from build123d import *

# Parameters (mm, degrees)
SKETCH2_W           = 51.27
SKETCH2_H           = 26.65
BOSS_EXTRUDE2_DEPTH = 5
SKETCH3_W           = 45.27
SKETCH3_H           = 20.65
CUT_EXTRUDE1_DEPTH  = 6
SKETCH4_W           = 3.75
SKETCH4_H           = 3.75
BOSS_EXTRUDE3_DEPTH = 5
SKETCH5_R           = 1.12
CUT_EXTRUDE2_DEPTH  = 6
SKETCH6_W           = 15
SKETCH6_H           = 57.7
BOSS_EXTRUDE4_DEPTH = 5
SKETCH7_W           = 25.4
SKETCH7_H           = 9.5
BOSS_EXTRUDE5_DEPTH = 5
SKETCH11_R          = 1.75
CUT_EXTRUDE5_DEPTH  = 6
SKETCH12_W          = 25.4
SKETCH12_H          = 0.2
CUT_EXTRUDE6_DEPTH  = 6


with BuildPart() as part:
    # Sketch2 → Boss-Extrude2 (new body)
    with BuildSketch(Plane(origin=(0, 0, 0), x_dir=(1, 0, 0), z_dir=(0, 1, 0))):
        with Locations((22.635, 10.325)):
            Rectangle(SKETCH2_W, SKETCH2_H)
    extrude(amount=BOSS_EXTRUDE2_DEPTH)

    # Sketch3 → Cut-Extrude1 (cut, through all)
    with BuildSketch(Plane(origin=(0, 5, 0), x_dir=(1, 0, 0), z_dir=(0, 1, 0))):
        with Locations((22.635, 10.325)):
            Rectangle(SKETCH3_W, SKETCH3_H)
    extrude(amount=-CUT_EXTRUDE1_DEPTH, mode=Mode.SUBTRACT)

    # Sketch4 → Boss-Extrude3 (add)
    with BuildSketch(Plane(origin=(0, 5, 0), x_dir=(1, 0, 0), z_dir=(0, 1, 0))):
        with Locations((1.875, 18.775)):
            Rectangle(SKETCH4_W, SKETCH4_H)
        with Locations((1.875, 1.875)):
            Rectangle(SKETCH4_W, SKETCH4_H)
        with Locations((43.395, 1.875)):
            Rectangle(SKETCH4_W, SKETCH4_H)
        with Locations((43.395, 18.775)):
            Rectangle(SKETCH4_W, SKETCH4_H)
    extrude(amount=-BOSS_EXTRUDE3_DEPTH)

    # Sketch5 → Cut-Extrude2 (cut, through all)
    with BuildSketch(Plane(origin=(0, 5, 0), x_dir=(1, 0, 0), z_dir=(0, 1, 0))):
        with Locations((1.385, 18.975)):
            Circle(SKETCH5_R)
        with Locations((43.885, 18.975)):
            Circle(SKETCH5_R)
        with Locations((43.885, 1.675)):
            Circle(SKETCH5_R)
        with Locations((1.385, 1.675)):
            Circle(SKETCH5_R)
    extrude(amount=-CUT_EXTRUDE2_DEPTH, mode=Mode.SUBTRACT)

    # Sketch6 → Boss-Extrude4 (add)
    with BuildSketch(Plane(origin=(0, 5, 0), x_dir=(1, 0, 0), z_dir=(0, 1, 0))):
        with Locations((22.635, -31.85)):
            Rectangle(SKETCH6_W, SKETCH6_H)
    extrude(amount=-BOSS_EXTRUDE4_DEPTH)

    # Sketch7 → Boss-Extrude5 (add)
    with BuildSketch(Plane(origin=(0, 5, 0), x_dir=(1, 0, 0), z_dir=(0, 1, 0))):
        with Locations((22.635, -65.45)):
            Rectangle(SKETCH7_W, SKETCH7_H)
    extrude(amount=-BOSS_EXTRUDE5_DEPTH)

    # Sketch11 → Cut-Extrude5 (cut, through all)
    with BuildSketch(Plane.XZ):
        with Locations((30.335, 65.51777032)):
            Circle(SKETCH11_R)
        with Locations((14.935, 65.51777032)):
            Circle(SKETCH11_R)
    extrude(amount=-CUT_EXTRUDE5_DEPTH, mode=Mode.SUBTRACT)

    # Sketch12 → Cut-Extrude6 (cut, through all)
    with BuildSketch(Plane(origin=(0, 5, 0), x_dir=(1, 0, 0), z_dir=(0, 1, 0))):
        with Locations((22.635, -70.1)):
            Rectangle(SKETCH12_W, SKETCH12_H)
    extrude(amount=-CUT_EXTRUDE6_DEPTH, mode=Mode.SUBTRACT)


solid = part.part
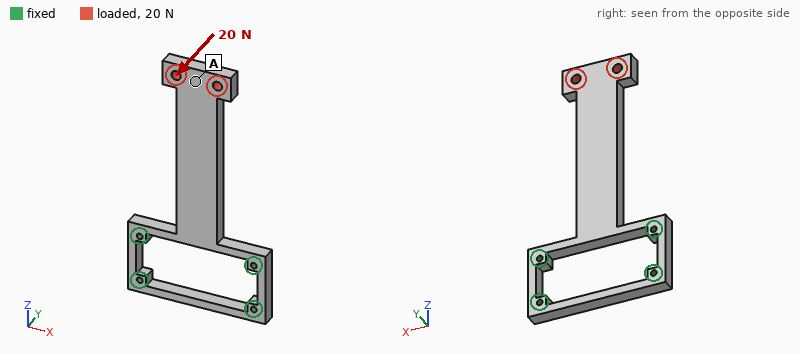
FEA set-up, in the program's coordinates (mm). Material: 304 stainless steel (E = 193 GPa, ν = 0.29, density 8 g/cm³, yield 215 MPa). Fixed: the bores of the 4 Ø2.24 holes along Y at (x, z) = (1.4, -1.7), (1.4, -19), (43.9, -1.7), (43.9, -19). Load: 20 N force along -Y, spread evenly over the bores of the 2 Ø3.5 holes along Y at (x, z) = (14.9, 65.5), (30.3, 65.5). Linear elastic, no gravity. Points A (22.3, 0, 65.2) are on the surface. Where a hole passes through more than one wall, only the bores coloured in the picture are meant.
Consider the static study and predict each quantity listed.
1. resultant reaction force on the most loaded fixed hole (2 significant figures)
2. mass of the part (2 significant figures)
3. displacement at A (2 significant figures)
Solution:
12 N
62 g
0.30 mm
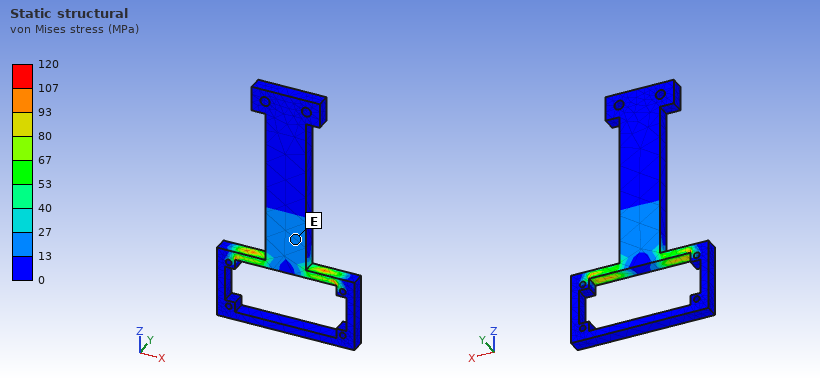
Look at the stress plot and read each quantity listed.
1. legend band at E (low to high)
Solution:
13 to 27 MPa
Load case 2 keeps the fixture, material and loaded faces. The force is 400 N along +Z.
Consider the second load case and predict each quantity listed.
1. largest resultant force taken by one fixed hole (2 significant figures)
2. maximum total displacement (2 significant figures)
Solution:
330 N
27 µm
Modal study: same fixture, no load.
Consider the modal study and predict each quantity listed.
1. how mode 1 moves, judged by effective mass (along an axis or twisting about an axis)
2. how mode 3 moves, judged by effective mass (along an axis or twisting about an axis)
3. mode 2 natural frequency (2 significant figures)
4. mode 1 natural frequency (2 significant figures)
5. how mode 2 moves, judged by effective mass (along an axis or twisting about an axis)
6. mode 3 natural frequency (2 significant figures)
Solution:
along Y
along Z
920 Hz
300 Hz
along X
2900 Hz
